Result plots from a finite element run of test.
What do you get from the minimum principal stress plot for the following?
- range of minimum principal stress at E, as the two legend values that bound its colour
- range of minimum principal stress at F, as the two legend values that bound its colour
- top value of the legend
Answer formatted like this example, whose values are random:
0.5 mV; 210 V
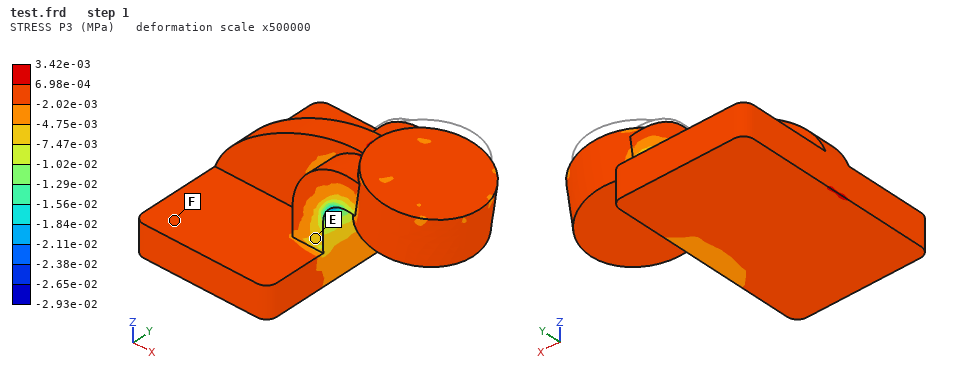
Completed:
-7.47e-03 to -4.75e-03 MPa; -2.02e-03 to 6.98e-04 MPa; 3.42e-03 MPa
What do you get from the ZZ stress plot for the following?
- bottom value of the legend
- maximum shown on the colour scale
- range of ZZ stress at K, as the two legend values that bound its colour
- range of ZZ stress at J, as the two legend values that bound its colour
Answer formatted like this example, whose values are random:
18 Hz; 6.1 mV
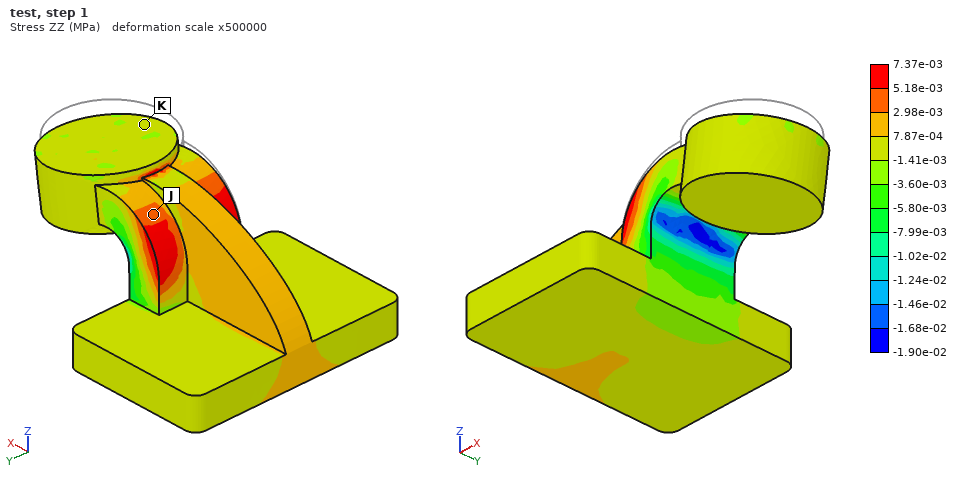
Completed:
-1.90e-02 MPa; 7.37e-03 MPa; -1.41e-03 to 7.87e-04 MPa; 2.98e-03 to 5.18e-03 MPa
